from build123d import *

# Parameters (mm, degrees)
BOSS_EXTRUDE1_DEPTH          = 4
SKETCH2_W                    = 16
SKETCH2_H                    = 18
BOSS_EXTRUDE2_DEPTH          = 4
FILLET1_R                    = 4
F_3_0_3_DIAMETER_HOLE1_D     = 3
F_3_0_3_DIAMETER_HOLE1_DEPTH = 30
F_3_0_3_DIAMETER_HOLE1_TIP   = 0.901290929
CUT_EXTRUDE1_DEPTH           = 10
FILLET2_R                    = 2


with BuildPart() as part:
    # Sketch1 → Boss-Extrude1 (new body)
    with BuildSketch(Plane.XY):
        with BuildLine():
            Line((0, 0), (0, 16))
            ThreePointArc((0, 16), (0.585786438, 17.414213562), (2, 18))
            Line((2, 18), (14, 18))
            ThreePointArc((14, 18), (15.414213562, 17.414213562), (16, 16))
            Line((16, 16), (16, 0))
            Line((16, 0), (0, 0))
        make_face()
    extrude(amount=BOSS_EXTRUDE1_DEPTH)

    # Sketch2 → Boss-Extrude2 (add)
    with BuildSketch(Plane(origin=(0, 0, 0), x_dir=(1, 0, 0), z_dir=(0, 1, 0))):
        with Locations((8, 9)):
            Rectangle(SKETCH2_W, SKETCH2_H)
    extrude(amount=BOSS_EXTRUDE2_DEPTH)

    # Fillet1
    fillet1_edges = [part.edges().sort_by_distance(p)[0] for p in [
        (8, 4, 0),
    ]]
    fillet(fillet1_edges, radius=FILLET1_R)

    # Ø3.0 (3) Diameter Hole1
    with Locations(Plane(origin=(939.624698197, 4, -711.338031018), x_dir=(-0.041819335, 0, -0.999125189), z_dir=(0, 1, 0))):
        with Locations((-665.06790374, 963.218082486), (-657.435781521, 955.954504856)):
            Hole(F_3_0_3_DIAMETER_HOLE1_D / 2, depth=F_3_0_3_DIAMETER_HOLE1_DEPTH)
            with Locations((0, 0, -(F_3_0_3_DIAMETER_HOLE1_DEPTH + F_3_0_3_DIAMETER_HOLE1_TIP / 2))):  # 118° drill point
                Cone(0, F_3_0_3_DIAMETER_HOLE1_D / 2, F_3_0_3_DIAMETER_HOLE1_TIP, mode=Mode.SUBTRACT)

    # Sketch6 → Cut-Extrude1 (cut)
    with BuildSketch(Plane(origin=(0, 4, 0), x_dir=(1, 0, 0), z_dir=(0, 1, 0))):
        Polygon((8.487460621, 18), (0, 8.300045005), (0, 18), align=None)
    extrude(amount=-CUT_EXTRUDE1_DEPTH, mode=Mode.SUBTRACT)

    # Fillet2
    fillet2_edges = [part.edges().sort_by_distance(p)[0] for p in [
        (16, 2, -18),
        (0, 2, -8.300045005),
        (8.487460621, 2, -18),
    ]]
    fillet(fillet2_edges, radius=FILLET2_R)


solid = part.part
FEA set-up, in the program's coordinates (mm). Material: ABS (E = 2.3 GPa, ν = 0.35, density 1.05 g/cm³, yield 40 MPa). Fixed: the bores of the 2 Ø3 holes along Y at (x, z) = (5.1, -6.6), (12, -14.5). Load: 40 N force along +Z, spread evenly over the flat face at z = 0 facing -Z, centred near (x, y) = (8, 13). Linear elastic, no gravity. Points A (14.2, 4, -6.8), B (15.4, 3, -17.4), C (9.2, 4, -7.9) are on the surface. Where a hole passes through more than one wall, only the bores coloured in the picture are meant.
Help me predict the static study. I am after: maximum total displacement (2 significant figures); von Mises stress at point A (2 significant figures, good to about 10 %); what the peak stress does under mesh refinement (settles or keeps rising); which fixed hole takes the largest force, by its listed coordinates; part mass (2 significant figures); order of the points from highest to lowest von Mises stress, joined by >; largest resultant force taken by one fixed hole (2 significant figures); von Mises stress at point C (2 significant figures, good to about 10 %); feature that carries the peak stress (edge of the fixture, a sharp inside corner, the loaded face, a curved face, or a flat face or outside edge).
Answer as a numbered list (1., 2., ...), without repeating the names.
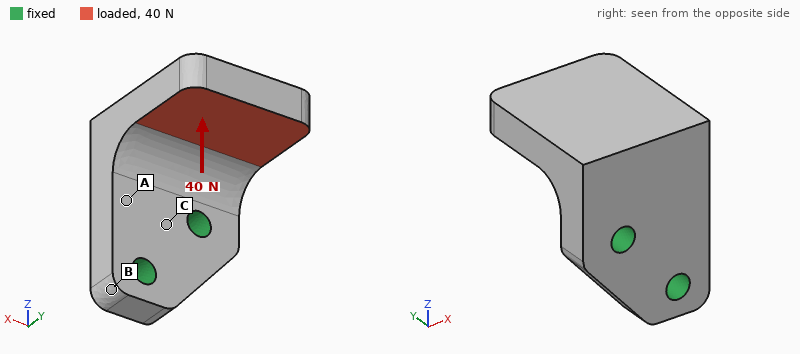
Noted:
1. 0.33 mm
2. 5.8 MPa
3. keeps rising
4. (5.1, -6.6)
5. 2.2 g
6. A > C > B
7. 31 N
8. 4.3 MPa
9. edge of the fixture
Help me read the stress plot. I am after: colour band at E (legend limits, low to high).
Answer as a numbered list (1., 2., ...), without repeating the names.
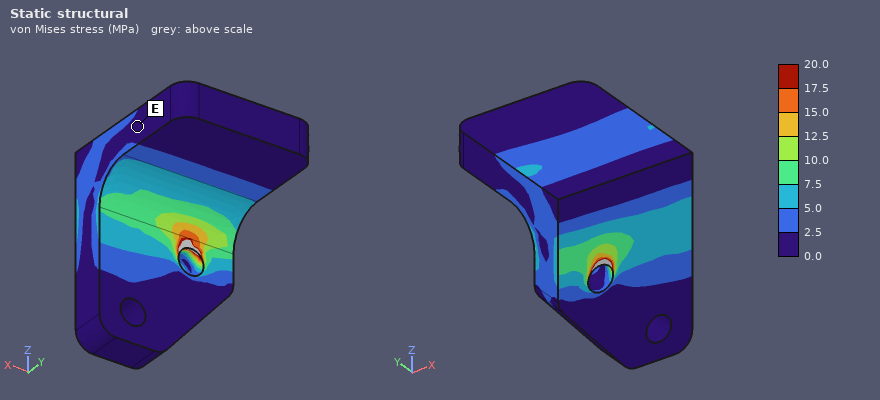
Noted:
1. 0.0 to 2.5 MPa
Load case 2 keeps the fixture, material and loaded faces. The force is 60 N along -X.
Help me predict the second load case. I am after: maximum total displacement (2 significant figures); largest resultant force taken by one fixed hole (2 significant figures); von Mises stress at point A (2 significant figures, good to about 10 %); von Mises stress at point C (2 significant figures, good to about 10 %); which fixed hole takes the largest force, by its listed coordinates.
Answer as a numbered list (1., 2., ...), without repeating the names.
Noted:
1. 0.31 mm
2. 76 N
3. 5.7 MPa
4. 6.5 MPa
5. (5.1, -6.6)
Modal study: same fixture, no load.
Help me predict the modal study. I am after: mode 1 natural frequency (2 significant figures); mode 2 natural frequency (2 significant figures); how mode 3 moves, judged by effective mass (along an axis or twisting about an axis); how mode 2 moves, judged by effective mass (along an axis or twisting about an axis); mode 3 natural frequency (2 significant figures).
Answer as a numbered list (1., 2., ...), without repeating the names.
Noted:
1. 2200 Hz
2. 3100 Hz
3. along Y
4. along X
5. 6800 Hz
